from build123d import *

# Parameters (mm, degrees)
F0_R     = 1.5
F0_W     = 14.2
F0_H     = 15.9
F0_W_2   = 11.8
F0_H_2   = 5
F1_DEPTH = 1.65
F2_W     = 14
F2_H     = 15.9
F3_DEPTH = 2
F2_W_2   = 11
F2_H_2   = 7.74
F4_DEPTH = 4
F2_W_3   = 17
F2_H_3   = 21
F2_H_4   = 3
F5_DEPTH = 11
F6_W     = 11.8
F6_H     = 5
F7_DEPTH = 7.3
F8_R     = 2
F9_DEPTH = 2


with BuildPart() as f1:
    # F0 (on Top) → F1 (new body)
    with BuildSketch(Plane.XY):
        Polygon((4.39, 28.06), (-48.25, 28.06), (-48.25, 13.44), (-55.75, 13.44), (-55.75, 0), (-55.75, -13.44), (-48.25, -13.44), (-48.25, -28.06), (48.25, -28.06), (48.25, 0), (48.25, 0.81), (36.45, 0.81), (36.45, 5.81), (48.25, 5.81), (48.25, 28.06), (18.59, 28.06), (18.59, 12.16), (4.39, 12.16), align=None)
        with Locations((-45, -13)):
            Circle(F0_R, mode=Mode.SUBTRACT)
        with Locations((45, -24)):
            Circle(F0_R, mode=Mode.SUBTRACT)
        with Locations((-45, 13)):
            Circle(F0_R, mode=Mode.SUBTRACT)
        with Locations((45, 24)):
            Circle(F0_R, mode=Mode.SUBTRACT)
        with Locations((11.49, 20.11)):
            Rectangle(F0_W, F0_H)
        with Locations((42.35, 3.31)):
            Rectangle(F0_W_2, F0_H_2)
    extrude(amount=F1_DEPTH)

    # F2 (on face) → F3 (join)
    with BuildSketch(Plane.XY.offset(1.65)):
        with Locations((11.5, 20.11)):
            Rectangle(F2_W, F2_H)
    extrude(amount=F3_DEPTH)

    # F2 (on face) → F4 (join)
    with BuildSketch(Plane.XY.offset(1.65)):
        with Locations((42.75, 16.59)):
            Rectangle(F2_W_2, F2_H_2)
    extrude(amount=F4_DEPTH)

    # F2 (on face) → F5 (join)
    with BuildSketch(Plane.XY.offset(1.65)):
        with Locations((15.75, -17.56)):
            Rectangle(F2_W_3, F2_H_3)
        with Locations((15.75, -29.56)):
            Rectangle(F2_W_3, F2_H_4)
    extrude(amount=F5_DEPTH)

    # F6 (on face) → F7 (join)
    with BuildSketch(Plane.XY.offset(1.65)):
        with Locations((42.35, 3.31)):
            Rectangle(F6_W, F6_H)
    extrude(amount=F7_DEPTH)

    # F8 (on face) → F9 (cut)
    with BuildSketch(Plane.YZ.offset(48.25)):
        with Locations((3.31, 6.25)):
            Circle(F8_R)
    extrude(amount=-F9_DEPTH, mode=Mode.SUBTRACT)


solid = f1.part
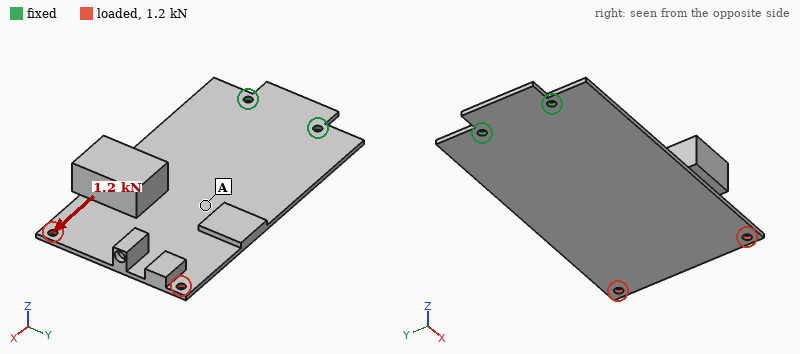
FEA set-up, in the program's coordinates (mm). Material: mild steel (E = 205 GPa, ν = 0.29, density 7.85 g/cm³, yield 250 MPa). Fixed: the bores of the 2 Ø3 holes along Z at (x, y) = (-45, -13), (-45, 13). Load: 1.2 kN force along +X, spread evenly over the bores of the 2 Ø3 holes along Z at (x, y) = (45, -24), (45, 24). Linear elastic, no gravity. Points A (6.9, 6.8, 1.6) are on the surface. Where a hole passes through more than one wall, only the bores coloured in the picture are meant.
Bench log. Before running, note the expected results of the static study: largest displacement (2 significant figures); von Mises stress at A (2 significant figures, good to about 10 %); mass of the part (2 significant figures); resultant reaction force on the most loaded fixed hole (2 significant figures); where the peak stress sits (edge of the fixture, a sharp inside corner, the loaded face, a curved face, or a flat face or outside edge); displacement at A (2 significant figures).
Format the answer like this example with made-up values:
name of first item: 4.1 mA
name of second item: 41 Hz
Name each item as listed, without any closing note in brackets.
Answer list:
largest displacement: 15 µm
von Mises stress at A: 9.1 MPa
mass of the part: 120 g
resultant reaction force on the most loaded fixed hole: 600 N
where the peak stress sits: the loaded face
displacement at A: 4.1 µm
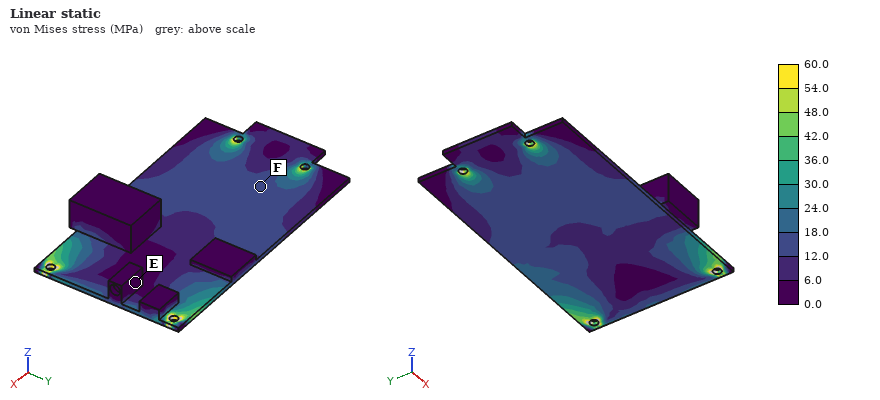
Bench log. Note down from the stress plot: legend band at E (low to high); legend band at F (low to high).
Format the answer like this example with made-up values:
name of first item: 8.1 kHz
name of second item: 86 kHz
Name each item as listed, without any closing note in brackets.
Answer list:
legend band at E: 0.0 to 6.0 MPa
legend band at F: 12.0 to 18.0 MPa
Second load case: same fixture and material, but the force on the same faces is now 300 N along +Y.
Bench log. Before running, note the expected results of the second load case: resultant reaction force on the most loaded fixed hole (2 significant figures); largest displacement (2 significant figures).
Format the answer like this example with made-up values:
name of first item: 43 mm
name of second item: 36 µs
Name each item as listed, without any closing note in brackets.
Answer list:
resultant reaction force on the most loaded fixed hole: 980 N
largest displacement: 41 µm
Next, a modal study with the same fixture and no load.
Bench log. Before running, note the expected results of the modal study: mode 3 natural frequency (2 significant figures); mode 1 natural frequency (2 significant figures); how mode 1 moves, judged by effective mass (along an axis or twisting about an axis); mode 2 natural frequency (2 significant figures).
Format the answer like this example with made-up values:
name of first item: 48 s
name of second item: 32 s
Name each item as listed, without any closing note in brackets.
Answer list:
mode 3 natural frequency: 890 Hz
mode 1 natural frequency: 110 Hz
how mode 1 moves, judged by effective mass: along Z
mode 2 natural frequency: 400 Hz
